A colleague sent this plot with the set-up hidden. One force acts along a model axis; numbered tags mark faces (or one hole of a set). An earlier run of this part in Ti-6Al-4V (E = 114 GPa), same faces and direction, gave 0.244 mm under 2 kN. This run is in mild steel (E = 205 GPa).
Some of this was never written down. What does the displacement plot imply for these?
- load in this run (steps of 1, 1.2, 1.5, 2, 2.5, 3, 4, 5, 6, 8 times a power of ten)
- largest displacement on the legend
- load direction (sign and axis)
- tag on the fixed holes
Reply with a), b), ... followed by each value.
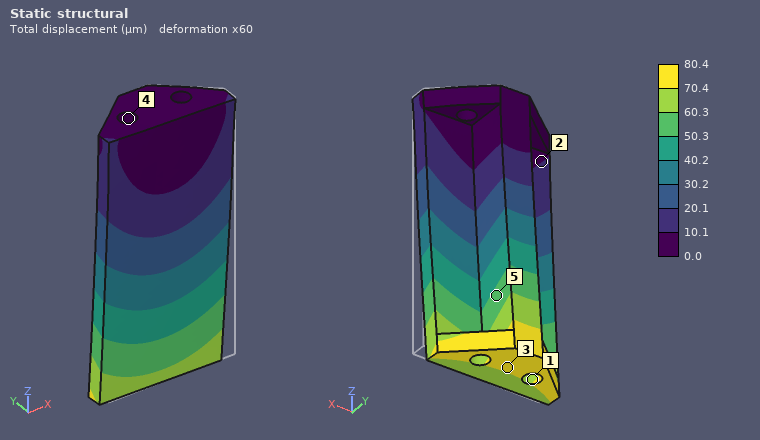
a) 1.2 kN
b) 80.4 µm
c) -X
d) 4
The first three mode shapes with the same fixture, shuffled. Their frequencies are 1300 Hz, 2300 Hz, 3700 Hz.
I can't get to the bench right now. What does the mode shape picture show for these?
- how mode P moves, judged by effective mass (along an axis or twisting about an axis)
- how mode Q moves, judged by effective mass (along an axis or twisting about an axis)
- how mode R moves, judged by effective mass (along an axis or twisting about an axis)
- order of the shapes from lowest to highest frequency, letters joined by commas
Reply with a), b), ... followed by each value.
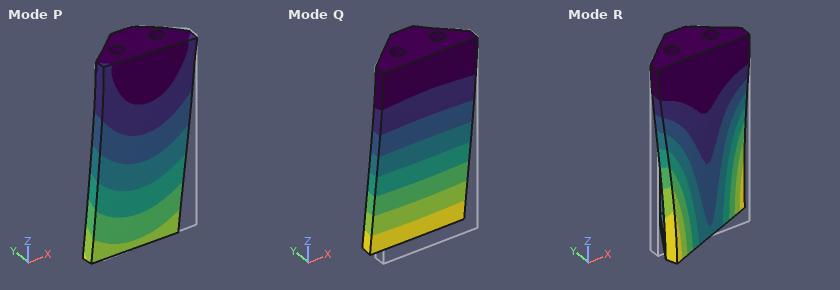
a) along X
b) along Y
c) twisting about Z
d) Q, P, R
